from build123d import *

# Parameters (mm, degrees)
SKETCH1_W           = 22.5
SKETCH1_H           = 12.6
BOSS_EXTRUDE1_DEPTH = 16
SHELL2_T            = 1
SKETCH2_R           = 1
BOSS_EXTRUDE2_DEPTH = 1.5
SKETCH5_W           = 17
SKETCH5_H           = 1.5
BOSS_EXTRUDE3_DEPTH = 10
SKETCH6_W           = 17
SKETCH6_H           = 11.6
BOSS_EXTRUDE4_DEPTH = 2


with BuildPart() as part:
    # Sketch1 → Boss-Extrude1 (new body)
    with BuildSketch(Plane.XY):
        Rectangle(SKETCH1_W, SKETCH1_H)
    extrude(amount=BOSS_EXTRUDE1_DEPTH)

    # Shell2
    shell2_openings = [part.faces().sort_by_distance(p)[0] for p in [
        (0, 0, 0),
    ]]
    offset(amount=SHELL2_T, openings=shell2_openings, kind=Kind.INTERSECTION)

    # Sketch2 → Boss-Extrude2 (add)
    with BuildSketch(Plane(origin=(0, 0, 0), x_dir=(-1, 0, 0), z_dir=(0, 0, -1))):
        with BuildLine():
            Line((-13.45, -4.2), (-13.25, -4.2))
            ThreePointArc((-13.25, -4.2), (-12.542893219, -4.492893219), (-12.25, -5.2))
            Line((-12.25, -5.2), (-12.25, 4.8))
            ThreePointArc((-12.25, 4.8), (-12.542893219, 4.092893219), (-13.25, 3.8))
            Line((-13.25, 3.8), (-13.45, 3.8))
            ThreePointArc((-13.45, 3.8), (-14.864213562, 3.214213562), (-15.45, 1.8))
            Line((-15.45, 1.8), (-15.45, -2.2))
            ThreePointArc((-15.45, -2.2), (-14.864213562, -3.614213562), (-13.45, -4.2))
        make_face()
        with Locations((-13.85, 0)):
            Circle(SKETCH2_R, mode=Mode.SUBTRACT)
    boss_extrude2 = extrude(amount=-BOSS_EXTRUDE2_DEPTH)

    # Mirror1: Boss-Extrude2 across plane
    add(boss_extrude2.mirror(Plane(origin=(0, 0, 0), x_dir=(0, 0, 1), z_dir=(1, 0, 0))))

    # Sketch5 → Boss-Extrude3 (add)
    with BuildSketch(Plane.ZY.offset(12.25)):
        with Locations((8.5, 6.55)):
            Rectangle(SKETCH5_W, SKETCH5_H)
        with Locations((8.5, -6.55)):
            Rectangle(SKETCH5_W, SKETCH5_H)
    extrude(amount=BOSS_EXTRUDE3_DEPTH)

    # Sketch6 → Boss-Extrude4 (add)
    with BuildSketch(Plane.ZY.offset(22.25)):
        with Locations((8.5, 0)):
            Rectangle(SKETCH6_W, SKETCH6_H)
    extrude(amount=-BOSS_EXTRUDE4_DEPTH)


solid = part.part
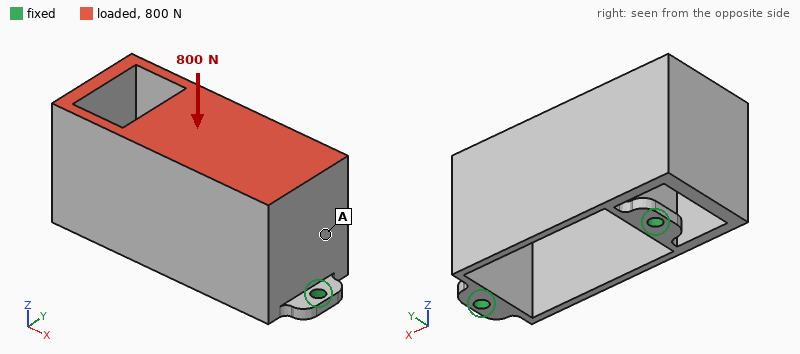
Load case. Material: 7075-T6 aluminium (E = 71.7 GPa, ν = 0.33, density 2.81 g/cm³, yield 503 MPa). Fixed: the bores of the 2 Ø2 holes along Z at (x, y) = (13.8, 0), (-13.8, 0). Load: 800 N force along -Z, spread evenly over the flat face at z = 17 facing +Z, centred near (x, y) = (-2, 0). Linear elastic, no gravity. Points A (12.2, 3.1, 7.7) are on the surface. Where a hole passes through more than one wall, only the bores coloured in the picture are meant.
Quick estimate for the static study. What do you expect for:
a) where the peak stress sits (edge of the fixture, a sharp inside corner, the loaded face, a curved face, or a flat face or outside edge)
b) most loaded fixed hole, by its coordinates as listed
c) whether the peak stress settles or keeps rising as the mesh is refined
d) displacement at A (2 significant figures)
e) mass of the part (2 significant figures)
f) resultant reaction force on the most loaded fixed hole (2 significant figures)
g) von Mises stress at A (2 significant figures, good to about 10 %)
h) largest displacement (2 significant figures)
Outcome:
edge of the fixture
(-13.8, 0)
keeps rising
9.7 µm
7.1 g
480 N
24 MPa
59 µm
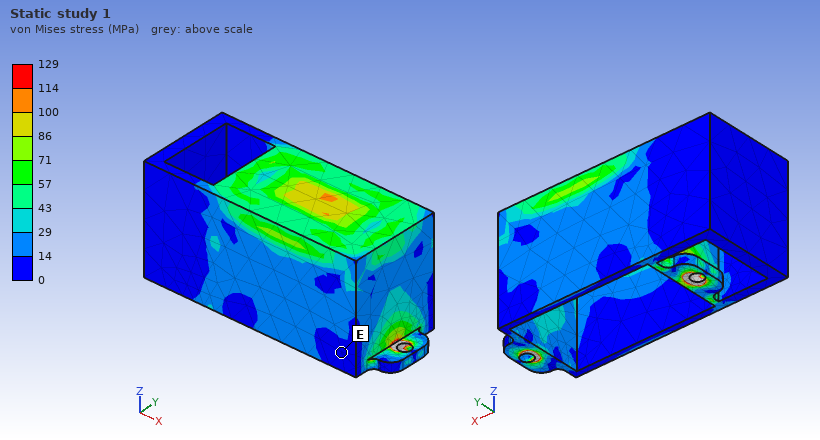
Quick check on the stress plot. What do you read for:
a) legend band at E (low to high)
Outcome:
0 to 14 MPa
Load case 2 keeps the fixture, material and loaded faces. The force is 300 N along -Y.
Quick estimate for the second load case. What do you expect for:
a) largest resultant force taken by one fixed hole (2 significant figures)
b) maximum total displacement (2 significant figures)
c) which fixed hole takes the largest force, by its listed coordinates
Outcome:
170 N
0.33 mm
(-13.8, 0)
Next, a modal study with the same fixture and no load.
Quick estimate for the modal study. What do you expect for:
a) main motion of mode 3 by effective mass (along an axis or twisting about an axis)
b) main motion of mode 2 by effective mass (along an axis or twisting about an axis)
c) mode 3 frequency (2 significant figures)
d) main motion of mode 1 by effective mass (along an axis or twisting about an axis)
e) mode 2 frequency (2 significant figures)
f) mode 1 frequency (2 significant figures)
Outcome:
along X
twisting about Z
7300 Hz
along Y
5800 Hz
2700 Hz
